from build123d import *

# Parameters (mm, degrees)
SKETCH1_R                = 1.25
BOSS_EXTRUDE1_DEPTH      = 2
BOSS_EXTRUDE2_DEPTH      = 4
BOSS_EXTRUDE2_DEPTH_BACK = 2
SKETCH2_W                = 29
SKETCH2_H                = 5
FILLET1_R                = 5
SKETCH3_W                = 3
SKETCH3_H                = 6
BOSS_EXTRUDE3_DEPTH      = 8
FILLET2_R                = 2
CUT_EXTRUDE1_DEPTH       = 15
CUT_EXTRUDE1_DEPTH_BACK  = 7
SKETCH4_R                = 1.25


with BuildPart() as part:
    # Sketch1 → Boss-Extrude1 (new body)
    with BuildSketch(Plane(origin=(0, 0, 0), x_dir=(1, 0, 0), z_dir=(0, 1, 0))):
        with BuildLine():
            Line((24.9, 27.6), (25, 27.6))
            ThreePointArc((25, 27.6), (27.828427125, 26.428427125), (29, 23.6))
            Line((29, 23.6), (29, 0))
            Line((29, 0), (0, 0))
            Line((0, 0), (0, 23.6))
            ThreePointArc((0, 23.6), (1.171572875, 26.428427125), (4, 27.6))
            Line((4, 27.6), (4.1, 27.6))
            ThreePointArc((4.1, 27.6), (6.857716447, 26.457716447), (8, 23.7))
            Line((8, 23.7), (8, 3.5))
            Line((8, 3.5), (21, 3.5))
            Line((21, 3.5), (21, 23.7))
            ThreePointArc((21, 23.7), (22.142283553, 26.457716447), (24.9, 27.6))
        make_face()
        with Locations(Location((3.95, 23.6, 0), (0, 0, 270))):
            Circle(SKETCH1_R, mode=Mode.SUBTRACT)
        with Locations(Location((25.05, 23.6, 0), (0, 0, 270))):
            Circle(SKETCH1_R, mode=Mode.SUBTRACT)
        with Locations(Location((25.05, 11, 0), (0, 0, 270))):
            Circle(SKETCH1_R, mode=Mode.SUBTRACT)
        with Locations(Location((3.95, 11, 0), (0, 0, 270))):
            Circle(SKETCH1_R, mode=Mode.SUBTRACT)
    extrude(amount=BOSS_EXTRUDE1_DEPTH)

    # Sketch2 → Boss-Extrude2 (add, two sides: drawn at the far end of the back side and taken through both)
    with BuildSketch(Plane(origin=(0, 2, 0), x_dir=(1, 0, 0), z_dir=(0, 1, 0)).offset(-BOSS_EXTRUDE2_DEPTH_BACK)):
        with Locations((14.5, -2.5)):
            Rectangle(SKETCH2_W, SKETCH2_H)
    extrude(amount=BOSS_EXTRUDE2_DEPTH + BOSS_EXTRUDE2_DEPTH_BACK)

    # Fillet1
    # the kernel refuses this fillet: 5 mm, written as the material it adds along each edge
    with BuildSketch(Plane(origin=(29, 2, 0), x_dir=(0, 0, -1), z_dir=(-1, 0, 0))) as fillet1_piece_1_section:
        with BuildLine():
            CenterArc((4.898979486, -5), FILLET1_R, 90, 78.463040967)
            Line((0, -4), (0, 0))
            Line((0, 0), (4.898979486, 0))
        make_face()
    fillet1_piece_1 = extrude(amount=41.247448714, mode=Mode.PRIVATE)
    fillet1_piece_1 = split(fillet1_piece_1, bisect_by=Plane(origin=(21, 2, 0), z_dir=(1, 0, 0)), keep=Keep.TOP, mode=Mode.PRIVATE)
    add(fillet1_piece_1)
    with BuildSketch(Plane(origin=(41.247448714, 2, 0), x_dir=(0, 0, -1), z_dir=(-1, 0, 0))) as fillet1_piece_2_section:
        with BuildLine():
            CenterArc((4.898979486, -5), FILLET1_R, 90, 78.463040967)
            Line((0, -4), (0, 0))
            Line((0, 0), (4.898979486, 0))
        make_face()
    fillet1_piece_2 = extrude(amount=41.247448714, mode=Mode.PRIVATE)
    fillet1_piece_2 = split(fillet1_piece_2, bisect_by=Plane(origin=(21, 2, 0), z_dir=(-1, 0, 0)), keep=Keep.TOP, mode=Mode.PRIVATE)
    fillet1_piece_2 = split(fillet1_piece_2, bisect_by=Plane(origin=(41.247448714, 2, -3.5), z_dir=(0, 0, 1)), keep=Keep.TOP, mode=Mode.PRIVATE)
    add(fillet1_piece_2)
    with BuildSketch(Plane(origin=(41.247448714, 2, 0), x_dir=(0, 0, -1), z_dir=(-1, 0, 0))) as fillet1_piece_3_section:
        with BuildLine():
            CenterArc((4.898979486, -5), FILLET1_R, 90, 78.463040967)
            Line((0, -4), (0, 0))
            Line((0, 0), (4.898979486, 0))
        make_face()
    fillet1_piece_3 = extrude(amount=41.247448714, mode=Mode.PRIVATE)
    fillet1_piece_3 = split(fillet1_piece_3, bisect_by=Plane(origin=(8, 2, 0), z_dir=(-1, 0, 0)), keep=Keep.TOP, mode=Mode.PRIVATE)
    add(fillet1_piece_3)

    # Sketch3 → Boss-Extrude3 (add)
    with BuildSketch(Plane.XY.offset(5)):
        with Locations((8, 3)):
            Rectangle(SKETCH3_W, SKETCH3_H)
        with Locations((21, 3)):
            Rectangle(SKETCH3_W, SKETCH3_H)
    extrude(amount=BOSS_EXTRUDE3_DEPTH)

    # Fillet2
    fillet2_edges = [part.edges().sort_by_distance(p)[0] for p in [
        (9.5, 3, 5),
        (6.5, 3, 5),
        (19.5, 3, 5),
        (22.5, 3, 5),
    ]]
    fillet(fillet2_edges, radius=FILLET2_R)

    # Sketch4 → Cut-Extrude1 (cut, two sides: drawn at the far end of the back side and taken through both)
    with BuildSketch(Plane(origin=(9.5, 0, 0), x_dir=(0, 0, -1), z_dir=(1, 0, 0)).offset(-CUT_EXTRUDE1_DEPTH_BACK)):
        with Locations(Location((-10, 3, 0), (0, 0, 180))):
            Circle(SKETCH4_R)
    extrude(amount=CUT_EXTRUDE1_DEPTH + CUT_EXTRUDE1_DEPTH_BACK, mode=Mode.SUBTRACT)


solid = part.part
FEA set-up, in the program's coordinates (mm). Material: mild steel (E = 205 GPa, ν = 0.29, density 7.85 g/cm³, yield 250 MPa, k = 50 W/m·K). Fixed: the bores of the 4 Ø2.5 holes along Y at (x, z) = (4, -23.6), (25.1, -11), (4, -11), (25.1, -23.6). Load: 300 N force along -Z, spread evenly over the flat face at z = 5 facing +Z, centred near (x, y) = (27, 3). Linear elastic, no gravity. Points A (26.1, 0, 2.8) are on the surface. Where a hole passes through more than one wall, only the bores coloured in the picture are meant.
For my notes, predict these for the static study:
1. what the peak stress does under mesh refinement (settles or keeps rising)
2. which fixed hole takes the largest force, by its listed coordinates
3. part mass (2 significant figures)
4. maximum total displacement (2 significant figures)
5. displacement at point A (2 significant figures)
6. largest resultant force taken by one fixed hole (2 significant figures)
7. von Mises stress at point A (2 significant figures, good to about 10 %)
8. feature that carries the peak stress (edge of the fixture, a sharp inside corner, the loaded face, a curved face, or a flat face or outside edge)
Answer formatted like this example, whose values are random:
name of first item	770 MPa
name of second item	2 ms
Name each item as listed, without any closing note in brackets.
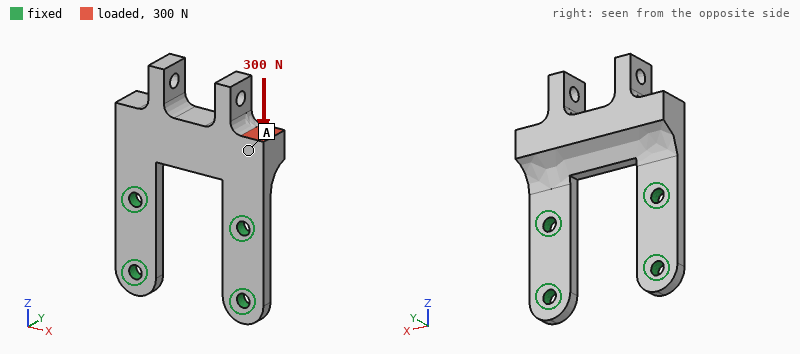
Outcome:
what the peak stress does under mesh refinement	keeps rising
which fixed hole takes the largest force, by its listed coordinates	(25.1, -11)
part mass	17 g
maximum total displacement	45 µm
displacement at point A	21 µm
largest resultant force taken by one fixed hole	290 N
von Mises stress at point A	12 MPa
feature that carries the peak stress	edge of the fixture
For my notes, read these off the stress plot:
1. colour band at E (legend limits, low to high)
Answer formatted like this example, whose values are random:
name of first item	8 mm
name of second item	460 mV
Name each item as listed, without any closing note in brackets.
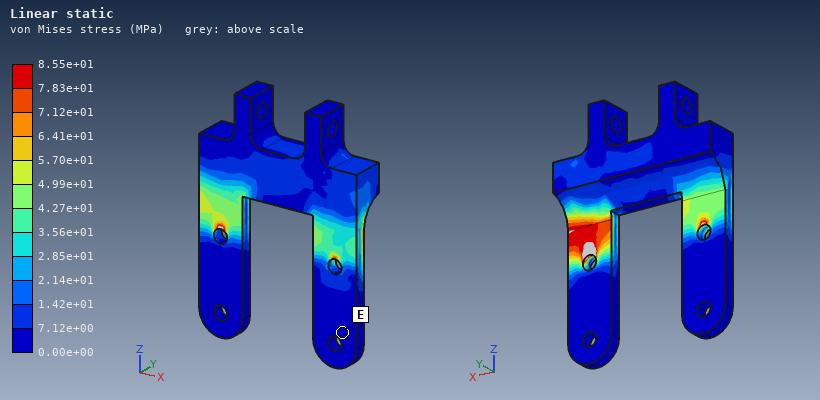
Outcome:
colour band at E	0.00e+00 to 7.12e+00 MPa
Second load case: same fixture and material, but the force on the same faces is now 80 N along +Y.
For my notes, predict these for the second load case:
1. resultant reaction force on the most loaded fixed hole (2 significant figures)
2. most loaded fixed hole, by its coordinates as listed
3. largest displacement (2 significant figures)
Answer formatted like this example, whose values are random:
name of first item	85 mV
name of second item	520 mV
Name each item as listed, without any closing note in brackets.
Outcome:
resultant reaction force on the most loaded fixed hole	85 N
most loaded fixed hole, by its coordinates as listed	(25.1, -11)
largest displacement	72 µm
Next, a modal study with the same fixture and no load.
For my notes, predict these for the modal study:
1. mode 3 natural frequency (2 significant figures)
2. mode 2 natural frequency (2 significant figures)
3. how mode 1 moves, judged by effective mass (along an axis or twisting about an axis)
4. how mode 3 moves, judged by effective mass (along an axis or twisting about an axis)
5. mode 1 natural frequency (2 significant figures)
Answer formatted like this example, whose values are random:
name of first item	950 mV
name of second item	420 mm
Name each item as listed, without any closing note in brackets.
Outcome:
mode 3 natural frequency	15 kHz
mode 2 natural frequency	9100 Hz
how mode 1 moves, judged by effective mass	along Y
how mode 3 moves, judged by effective mass	along X
mode 1 natural frequency	2400 Hz
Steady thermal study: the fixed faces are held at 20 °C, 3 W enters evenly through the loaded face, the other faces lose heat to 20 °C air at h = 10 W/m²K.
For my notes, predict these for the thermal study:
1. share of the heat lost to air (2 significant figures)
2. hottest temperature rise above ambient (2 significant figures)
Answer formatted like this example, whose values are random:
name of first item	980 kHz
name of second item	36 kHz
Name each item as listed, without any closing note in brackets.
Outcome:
share of the heat lost to air	6.9 %
hottest temperature rise above ambient	30 K
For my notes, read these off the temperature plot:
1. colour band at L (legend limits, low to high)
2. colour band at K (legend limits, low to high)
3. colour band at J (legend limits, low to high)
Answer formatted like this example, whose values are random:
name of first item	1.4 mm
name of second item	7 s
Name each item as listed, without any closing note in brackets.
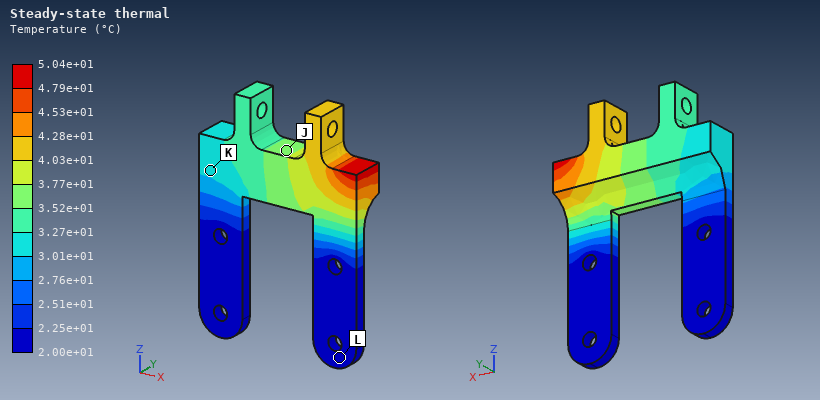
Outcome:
colour band at L	2.00e+01 to 2.25e+01 °C
colour band at K	3.01e+01 to 3.27e+01 °C
colour band at J	3.52e+01 to 3.77e+01 °C
